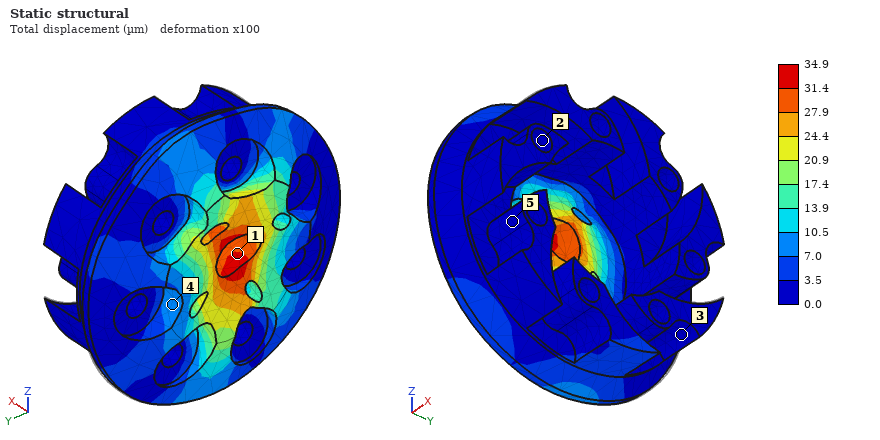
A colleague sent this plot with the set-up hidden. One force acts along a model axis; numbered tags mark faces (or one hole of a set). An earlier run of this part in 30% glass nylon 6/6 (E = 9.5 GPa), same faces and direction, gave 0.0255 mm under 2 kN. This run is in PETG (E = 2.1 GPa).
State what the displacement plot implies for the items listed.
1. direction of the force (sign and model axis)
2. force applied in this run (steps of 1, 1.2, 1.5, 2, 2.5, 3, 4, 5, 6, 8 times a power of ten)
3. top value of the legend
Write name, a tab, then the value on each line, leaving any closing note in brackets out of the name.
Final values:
direction of the force	+Z
force applied in this run	600 N
top value of the legend	34.9 µm
